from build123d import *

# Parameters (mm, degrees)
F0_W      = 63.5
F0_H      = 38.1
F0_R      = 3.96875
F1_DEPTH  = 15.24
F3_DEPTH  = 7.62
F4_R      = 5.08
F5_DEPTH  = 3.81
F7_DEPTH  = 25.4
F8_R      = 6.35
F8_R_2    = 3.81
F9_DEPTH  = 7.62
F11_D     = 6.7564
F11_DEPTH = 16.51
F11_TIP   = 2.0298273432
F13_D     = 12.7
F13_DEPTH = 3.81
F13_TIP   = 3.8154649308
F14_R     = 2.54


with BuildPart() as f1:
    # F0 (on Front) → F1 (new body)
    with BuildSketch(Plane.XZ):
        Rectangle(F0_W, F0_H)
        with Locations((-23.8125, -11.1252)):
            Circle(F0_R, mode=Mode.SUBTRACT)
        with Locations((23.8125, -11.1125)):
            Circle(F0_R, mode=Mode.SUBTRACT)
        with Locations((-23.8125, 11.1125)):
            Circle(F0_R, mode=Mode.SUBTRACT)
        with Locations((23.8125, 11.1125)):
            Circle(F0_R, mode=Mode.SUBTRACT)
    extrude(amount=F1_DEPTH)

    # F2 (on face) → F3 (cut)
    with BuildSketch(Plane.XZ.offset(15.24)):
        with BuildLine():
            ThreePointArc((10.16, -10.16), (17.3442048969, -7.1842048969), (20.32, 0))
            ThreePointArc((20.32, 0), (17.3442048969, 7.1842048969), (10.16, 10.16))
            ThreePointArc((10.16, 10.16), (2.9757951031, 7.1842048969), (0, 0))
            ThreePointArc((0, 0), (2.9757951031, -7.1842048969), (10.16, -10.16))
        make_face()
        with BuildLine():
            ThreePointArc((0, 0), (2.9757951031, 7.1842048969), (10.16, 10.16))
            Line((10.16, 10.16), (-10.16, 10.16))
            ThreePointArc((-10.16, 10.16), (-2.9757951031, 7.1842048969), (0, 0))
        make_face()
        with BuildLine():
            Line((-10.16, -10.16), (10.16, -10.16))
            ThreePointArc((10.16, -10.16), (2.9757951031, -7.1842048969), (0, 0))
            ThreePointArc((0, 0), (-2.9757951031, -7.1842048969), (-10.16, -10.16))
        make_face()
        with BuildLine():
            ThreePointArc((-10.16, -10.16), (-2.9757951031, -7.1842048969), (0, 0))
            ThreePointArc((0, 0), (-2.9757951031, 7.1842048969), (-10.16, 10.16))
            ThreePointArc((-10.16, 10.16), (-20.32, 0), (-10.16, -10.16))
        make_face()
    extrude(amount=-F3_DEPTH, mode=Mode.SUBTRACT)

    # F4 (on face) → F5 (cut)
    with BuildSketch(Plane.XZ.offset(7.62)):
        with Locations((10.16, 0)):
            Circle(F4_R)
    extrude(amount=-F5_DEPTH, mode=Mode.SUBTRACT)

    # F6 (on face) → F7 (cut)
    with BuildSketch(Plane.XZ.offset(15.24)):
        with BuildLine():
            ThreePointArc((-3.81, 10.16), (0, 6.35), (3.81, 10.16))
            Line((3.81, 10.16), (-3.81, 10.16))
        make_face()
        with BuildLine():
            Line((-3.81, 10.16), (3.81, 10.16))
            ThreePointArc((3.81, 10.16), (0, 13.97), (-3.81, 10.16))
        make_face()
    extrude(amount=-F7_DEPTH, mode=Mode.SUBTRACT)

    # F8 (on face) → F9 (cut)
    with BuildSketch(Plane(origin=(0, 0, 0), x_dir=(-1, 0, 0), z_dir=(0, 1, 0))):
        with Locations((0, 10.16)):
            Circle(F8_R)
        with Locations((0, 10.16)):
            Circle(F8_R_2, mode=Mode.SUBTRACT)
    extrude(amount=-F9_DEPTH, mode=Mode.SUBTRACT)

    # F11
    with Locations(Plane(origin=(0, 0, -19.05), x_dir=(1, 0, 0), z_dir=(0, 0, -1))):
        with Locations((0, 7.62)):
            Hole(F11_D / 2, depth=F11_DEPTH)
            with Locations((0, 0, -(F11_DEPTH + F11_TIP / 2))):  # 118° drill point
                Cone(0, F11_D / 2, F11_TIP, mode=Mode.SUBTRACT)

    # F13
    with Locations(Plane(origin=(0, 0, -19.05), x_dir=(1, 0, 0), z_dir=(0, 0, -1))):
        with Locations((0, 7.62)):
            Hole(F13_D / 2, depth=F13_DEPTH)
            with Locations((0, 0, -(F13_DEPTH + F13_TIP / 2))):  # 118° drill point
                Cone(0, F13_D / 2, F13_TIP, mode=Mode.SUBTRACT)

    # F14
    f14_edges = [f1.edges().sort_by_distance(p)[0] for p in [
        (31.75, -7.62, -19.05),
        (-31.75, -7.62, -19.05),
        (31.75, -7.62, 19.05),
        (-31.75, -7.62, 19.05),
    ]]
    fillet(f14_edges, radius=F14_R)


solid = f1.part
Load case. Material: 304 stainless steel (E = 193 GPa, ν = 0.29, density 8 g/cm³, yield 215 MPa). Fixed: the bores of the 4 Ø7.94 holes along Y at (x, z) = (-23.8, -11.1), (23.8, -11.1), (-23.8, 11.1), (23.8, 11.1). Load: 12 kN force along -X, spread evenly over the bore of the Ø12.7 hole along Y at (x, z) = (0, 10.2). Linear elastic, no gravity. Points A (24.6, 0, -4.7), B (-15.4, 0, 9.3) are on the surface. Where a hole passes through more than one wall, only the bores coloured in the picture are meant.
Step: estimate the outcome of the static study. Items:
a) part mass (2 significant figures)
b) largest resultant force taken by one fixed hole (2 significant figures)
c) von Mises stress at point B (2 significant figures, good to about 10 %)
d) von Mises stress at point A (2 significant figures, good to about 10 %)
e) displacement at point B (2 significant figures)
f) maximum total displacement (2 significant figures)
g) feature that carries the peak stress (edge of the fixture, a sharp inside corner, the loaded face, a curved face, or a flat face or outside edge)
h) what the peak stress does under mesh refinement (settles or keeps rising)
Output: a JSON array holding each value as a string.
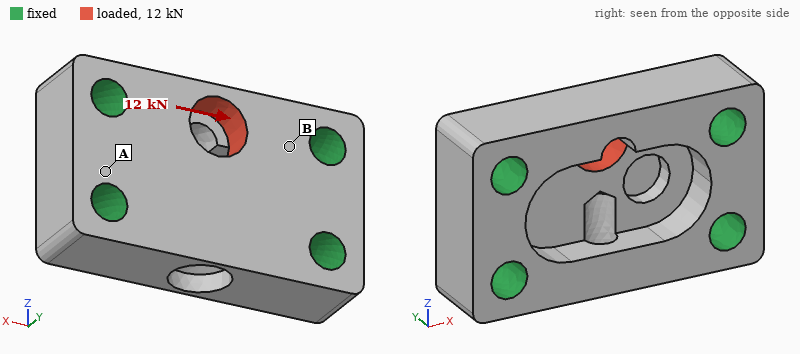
["210 g", "4.9 kN", "38 MPa", "8.4 MPa", "0.98 µm", "4.1 µm", "a sharp inside corner", "keeps rising"]
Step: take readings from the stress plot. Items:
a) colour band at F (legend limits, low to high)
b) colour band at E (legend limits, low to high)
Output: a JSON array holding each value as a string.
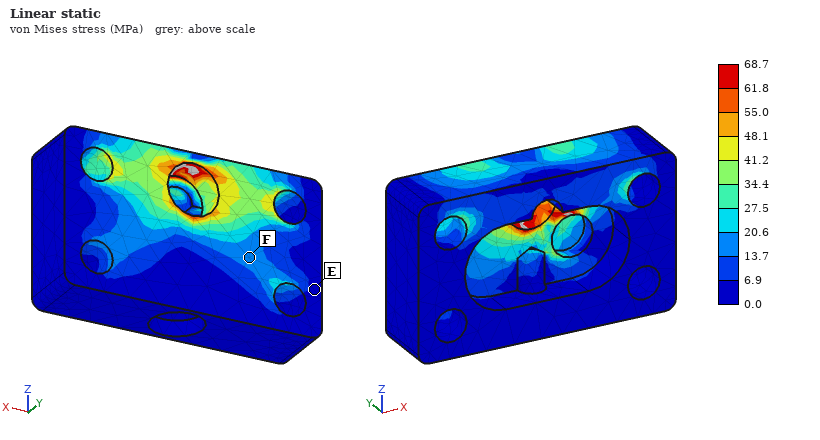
["13.7 to 20.6 MPa", "0.0 to 6.9 MPa"]
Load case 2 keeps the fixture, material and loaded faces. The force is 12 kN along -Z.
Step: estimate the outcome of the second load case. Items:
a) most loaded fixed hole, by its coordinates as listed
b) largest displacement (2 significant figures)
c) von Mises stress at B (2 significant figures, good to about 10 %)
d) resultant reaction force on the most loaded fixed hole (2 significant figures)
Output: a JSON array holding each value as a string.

["(-23.8, -11.1)", "17 µm", "45 MPa", "3.9 kN"]
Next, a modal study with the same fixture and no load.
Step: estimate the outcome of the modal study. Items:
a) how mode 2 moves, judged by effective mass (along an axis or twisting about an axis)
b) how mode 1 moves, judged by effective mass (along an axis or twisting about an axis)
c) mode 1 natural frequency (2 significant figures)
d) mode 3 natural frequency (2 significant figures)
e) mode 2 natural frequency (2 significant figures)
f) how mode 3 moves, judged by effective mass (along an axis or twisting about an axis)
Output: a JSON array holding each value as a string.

["along Z", "along Y", "26 kHz", "32 kHz", "29 kHz", "along Z"]
